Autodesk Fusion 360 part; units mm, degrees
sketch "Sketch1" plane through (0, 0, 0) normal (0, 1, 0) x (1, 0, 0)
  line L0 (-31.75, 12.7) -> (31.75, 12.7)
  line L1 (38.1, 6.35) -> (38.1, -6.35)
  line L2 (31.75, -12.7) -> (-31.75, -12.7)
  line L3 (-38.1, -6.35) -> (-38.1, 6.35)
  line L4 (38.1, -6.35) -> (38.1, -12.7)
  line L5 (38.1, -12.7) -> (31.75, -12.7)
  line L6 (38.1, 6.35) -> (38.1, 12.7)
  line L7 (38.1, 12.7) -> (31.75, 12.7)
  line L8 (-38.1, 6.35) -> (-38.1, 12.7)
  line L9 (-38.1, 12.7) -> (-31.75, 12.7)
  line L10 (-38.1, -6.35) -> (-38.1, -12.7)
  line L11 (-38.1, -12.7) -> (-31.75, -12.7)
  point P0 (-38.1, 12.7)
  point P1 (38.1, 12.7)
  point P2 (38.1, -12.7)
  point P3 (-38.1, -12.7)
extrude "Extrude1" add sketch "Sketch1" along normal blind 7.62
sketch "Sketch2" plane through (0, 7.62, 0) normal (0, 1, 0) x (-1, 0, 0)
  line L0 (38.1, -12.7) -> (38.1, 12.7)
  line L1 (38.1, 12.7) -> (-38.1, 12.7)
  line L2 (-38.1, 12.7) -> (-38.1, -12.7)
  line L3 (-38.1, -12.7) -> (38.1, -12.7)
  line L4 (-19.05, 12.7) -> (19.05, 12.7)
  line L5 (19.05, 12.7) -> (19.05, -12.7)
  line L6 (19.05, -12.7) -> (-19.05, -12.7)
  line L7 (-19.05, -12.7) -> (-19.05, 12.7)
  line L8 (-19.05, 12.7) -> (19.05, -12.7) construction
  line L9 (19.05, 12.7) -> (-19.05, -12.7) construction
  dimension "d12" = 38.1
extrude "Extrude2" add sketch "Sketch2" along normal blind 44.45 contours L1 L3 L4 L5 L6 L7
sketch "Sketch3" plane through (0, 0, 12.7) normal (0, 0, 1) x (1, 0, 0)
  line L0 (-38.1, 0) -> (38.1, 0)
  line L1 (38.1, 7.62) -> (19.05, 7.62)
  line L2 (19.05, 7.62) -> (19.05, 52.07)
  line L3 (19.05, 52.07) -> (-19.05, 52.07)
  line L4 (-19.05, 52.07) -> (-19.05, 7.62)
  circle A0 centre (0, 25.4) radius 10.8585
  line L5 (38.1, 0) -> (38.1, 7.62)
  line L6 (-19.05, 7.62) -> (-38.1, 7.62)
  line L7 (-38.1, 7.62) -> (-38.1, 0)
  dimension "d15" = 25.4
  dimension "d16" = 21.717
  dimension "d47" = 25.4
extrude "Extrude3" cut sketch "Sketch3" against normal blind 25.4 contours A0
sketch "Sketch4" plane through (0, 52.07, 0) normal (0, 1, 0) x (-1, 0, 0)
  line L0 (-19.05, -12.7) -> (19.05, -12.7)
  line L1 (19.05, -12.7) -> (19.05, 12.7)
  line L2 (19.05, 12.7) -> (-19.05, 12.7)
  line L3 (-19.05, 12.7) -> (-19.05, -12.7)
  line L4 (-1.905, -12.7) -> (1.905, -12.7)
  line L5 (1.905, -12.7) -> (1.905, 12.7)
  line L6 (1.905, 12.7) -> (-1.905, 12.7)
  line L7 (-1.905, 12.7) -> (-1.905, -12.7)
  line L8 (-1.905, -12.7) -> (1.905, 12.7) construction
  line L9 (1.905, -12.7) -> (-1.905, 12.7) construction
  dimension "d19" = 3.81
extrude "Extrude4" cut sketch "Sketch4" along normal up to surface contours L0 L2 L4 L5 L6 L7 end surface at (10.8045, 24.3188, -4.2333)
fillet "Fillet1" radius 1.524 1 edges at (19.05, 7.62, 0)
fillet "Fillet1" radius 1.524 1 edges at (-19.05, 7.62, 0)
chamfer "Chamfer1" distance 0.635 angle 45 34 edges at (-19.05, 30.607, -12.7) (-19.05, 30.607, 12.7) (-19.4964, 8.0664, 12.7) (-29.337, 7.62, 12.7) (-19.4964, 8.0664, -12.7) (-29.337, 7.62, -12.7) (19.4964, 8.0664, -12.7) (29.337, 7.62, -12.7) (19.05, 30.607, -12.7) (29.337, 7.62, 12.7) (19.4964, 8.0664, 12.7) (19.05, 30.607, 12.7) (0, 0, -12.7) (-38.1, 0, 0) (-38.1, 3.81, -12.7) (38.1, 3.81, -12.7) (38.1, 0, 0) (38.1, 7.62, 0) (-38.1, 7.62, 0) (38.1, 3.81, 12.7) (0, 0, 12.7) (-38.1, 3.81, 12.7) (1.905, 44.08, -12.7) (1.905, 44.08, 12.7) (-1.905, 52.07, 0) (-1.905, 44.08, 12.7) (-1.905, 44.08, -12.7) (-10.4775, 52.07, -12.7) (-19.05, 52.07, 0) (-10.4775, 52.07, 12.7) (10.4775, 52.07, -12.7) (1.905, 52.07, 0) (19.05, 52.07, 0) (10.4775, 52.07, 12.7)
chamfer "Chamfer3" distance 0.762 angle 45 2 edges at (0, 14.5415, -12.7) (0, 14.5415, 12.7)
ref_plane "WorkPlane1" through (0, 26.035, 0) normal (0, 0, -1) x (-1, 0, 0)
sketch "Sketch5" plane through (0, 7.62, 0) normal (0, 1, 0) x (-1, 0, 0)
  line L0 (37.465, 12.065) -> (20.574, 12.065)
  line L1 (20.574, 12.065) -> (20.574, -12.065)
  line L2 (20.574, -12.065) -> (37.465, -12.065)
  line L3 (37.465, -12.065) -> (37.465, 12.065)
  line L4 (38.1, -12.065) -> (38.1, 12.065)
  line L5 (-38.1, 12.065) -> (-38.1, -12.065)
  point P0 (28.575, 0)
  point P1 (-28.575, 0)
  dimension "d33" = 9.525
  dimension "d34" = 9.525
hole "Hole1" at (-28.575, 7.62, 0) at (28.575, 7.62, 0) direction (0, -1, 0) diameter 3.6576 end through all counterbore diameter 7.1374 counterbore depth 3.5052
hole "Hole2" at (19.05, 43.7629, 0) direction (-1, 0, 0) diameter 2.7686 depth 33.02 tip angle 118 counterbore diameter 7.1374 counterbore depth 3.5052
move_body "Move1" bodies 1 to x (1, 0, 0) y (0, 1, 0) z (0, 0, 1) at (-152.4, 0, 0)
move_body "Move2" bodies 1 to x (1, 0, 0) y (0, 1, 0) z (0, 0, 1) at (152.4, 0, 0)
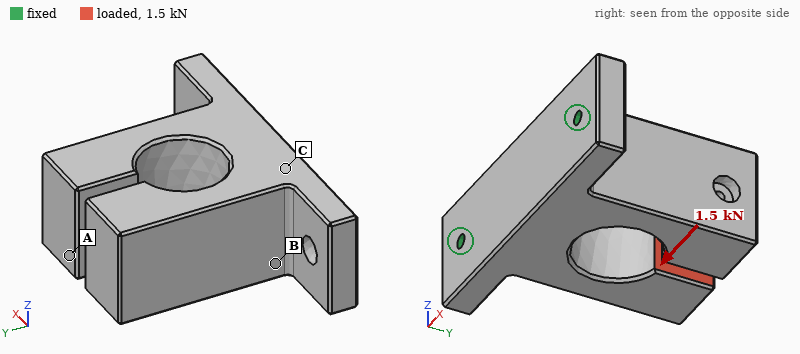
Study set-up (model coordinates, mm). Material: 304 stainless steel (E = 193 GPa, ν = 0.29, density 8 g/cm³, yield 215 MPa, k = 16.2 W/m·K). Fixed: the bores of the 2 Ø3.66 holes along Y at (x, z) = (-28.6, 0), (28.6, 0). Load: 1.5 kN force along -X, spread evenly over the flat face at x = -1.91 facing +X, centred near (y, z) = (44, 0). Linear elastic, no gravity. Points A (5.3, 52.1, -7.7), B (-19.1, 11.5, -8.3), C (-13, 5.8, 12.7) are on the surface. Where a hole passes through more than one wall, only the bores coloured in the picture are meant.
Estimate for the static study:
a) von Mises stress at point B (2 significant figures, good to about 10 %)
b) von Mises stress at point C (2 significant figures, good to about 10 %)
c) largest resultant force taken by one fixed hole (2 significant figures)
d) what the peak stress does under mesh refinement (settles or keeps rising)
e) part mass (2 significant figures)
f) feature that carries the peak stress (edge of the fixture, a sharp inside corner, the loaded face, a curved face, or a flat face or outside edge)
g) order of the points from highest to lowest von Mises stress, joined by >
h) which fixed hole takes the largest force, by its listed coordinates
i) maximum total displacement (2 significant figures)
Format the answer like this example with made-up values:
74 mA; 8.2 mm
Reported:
52 MPa; 33 MPa; 1.8 kN; keeps rising; 370 g; edge of the fixture; B > C > A; (28.6, 0); 83 µm
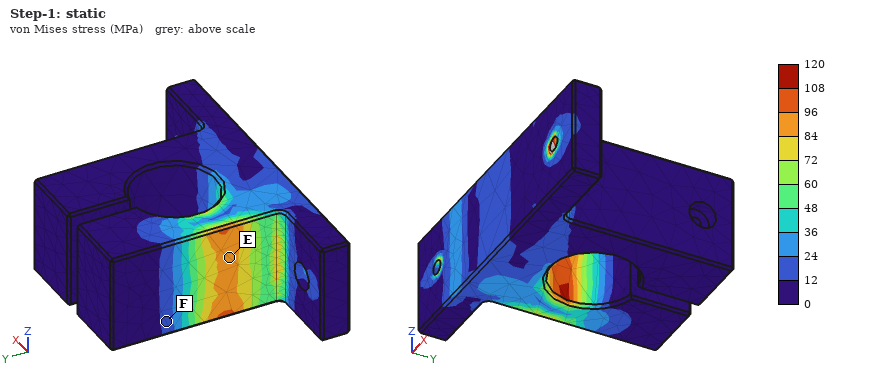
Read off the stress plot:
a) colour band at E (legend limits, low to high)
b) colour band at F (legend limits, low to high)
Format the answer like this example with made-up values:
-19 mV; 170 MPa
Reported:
84 to 96 MPa; 12 to 24 MPa
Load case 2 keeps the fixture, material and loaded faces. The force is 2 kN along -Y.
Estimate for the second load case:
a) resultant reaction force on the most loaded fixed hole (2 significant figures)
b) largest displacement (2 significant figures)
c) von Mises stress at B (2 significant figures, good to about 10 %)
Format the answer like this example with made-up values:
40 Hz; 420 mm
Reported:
1.6 kN; 63 µm; 16 MPa
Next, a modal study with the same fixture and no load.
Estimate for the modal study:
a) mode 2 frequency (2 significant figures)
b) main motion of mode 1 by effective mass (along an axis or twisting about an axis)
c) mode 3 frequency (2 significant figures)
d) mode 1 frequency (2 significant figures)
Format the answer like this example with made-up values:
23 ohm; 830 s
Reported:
3100 Hz; along Z; 3100 Hz; 1200 Hz
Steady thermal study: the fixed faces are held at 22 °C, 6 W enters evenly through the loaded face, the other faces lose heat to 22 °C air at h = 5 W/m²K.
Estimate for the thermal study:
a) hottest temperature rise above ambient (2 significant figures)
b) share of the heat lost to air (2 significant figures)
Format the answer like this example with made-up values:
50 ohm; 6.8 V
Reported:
68 K; 22 %
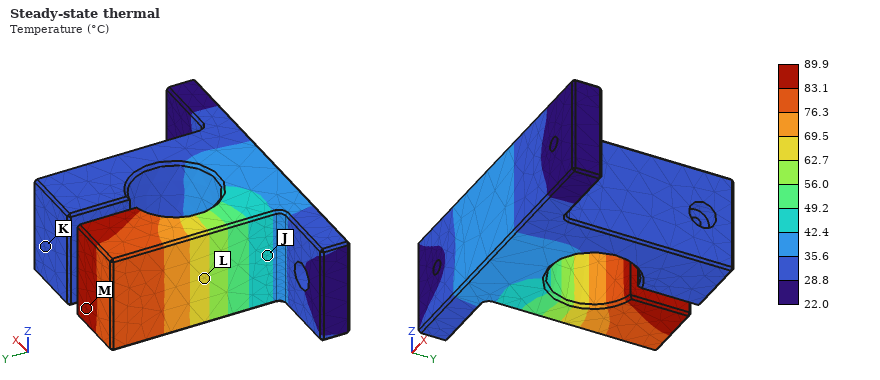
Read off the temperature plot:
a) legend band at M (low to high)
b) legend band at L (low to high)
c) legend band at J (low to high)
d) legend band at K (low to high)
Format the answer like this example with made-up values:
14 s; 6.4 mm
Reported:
83.1 to 89.9 °C; 62.7 to 69.5 °C; 42.4 to 49.2 °C; 28.8 to 35.6 °C
